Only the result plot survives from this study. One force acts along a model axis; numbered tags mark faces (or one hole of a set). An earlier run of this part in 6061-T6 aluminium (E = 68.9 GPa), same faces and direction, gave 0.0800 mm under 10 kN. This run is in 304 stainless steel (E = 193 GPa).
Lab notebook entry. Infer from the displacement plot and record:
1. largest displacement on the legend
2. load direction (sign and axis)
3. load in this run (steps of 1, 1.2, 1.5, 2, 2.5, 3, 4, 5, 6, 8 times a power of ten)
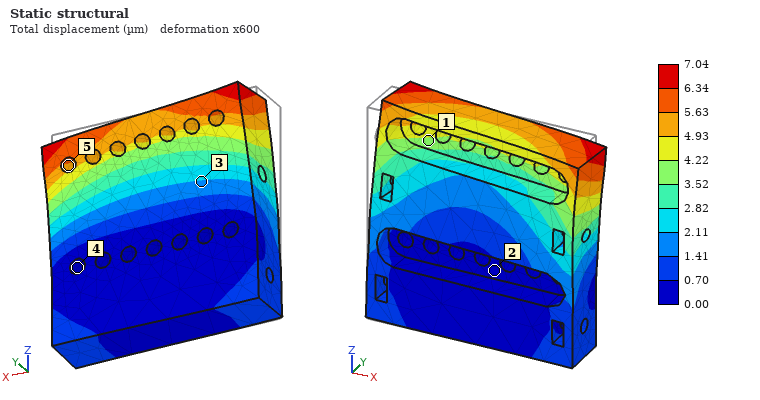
7.04 µm
+X
2.5 kN
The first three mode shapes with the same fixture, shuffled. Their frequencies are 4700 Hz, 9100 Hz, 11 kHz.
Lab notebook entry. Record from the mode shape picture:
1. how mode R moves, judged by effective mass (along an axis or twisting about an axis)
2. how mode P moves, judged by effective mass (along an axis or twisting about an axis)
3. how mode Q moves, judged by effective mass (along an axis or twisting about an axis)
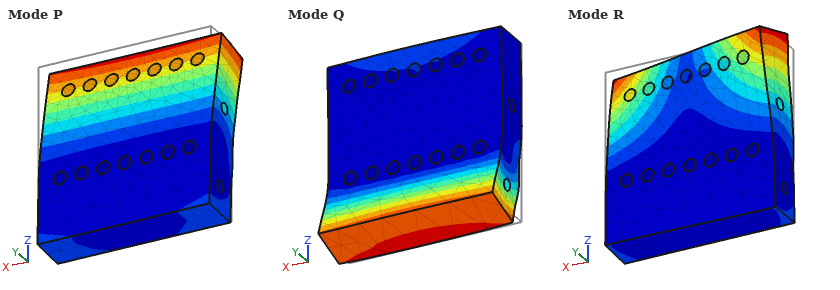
twisting about Z
along Y
along Y
